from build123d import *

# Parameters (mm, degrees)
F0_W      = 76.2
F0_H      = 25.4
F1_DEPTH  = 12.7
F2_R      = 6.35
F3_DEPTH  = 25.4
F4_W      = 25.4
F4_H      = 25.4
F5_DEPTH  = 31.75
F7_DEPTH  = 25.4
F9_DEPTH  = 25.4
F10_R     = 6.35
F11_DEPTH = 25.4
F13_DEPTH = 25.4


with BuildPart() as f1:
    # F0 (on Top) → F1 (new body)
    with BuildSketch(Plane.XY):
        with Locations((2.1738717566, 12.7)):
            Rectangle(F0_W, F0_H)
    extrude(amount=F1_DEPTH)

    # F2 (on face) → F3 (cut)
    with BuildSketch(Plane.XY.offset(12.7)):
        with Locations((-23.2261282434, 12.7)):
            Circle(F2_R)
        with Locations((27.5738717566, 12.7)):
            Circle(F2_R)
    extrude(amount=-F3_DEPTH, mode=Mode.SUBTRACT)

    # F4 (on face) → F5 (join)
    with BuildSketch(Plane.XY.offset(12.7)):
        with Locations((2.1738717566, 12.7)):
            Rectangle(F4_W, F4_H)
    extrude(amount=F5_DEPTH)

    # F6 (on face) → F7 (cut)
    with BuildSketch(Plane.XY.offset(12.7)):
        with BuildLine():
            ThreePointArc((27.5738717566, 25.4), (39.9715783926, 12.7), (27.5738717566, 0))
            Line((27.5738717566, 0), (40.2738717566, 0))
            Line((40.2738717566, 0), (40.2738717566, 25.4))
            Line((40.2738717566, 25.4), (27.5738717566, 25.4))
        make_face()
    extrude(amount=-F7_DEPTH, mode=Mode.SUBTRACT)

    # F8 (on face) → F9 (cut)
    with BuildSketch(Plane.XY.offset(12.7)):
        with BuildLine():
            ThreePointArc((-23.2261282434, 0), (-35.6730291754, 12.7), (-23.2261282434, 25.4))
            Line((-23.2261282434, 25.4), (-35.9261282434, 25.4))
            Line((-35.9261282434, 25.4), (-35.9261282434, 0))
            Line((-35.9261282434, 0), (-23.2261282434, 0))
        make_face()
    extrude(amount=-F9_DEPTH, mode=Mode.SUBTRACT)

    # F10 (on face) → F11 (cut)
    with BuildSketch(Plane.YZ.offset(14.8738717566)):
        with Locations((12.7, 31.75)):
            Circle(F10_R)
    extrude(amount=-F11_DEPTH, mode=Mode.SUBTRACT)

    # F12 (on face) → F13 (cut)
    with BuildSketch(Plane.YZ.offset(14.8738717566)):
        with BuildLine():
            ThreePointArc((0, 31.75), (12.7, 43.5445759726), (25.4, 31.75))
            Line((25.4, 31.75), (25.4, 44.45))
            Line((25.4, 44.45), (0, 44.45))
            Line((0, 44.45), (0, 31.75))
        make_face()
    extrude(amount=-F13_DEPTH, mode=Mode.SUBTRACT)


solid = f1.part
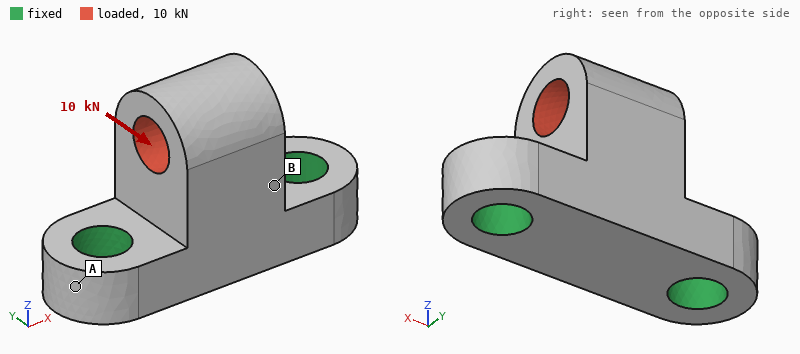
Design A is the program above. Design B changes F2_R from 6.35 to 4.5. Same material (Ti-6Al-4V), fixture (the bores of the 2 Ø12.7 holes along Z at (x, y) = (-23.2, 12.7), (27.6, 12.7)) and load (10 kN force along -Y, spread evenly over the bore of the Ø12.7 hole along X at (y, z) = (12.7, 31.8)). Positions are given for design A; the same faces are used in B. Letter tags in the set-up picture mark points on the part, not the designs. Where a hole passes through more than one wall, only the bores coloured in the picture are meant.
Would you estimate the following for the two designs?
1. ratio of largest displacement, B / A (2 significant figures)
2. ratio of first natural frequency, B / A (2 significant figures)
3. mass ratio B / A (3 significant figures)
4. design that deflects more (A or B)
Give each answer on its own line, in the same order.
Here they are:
1.2
0.90
1.05
B
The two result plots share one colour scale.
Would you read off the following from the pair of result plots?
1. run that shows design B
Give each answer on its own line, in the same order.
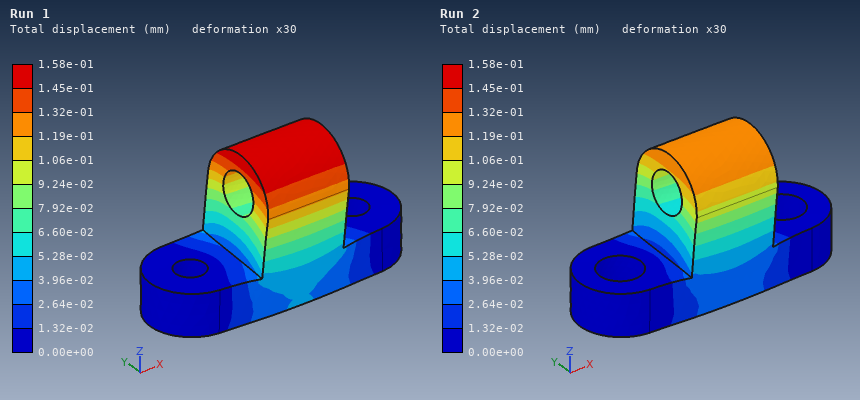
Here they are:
Run 1
